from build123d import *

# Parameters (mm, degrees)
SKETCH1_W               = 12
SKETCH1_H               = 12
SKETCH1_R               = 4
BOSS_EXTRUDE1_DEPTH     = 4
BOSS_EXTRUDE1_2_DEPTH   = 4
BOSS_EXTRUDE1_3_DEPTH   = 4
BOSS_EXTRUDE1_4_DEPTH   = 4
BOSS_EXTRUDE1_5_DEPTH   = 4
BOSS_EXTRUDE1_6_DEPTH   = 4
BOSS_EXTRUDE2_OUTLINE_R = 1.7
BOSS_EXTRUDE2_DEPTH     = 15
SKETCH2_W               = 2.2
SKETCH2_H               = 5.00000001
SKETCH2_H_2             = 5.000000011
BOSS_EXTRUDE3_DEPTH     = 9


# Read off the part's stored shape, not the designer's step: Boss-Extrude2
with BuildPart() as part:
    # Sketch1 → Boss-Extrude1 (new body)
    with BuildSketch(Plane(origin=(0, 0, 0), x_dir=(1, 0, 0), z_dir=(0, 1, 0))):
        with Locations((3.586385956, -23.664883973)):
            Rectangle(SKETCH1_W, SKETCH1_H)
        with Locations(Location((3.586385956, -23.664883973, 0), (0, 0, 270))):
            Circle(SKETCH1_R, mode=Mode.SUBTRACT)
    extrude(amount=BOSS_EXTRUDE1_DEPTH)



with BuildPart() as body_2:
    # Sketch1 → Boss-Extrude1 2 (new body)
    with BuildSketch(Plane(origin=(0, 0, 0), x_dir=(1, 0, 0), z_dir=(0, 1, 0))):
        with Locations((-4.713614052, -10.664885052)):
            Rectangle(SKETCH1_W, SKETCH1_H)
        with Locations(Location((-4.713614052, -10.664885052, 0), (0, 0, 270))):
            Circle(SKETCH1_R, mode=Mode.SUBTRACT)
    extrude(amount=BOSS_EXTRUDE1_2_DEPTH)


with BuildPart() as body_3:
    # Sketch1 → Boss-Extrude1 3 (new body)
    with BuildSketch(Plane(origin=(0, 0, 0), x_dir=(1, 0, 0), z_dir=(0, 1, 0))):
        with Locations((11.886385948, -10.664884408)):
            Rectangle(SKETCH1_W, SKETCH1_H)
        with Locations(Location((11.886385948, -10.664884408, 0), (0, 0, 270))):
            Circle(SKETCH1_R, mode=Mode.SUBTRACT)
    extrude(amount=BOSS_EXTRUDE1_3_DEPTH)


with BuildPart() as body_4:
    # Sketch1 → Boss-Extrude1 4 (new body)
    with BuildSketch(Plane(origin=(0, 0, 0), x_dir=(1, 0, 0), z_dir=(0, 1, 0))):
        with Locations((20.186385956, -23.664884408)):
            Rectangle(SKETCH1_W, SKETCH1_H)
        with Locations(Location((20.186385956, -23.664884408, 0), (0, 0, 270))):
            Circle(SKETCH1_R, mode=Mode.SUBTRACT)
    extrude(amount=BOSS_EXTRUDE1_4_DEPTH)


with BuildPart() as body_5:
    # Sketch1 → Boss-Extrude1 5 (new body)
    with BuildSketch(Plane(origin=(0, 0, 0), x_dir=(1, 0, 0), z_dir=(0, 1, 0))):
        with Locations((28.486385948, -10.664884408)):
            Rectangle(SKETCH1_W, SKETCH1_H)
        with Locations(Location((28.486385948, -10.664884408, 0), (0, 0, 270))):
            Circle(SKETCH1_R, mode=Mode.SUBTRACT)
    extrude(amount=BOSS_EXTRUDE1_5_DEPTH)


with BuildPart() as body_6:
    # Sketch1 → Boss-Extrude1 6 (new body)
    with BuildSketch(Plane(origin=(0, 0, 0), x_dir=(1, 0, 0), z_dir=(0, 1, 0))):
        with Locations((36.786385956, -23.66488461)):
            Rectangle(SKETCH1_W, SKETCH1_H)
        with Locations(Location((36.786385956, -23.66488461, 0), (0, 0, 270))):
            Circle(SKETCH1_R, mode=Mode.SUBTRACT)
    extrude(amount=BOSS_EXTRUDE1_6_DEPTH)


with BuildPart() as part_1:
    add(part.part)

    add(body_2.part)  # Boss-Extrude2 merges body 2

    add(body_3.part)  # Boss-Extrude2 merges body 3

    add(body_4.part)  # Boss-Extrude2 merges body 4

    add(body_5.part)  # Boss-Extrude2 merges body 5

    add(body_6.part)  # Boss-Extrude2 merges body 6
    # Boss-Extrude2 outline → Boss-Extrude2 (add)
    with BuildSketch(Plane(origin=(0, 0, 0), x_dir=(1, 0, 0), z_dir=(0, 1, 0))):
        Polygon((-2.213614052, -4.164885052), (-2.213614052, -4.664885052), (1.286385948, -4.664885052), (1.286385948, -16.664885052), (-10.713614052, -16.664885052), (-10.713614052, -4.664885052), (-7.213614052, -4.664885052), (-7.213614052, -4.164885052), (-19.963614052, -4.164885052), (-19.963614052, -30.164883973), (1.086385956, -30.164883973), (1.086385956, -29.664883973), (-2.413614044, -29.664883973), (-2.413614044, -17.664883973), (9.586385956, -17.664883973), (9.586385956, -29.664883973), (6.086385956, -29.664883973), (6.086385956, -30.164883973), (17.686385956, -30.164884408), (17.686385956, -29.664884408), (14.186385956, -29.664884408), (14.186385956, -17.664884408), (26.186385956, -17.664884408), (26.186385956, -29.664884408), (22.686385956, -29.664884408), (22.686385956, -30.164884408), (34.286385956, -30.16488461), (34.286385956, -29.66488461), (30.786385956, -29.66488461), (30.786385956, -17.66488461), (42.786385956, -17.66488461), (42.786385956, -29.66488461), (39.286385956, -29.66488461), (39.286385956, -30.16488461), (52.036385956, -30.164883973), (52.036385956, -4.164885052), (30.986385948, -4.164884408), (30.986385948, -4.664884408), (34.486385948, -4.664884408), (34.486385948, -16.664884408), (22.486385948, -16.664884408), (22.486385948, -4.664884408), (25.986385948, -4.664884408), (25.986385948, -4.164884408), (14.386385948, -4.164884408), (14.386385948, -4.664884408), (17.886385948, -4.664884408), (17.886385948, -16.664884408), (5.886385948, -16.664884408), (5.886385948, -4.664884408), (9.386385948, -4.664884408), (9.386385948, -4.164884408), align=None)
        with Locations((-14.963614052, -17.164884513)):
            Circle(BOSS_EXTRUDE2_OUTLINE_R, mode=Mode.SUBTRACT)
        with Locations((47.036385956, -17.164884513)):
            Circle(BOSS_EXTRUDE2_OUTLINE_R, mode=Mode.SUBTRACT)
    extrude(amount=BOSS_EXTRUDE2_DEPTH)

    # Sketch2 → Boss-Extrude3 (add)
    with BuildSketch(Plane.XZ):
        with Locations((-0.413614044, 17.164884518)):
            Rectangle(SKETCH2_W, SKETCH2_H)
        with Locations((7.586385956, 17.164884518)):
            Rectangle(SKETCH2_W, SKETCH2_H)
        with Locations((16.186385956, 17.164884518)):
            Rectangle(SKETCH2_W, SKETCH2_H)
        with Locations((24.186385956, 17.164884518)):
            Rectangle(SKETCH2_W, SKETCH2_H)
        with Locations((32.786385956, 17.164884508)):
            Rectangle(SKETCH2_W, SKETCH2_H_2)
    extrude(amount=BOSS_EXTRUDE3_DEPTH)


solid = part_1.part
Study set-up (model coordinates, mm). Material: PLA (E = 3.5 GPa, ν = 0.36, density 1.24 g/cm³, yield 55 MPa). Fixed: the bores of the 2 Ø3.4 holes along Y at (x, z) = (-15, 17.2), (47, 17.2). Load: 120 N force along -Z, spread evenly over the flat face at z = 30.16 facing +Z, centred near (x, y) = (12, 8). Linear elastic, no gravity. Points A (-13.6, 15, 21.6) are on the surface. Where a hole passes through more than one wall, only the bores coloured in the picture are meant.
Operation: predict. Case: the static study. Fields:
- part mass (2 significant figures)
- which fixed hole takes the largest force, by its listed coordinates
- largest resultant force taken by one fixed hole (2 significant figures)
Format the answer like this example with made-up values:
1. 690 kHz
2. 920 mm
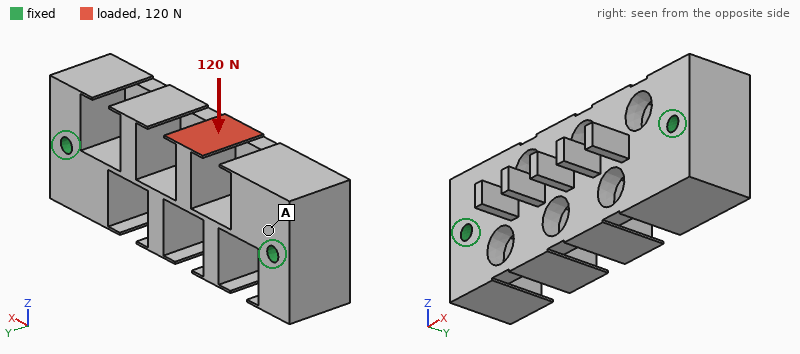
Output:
1. 22 g
2. (-15, 17.2)
3. 70 N
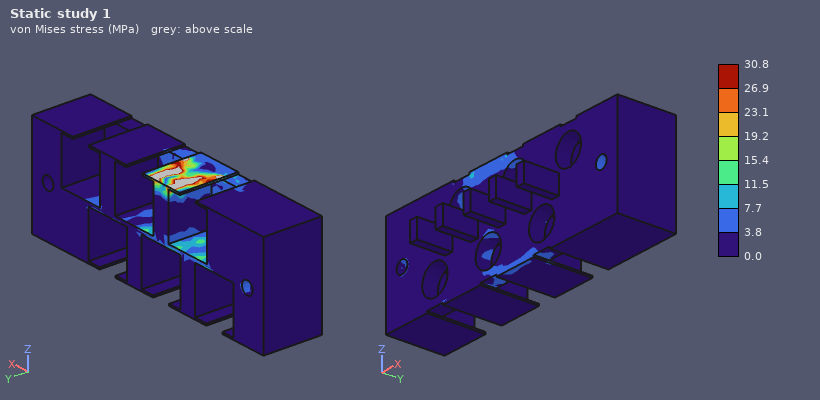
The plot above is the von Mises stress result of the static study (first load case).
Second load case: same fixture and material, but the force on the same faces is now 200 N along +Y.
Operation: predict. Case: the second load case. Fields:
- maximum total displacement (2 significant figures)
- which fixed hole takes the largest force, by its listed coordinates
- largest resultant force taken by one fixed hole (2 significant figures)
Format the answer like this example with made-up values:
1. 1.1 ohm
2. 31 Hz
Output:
1. 0.49 mm
2. (-15, 17.2)
3. 130 N
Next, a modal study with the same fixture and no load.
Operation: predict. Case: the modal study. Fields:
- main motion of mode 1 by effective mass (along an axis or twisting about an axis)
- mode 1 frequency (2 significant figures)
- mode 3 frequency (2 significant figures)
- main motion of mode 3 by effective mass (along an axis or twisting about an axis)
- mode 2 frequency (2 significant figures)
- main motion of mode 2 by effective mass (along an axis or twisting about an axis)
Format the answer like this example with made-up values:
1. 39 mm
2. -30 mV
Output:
1. along Z
2. 2800 Hz
3. 3400 Hz
4. along Z
5. 3000 Hz
6. along Y
